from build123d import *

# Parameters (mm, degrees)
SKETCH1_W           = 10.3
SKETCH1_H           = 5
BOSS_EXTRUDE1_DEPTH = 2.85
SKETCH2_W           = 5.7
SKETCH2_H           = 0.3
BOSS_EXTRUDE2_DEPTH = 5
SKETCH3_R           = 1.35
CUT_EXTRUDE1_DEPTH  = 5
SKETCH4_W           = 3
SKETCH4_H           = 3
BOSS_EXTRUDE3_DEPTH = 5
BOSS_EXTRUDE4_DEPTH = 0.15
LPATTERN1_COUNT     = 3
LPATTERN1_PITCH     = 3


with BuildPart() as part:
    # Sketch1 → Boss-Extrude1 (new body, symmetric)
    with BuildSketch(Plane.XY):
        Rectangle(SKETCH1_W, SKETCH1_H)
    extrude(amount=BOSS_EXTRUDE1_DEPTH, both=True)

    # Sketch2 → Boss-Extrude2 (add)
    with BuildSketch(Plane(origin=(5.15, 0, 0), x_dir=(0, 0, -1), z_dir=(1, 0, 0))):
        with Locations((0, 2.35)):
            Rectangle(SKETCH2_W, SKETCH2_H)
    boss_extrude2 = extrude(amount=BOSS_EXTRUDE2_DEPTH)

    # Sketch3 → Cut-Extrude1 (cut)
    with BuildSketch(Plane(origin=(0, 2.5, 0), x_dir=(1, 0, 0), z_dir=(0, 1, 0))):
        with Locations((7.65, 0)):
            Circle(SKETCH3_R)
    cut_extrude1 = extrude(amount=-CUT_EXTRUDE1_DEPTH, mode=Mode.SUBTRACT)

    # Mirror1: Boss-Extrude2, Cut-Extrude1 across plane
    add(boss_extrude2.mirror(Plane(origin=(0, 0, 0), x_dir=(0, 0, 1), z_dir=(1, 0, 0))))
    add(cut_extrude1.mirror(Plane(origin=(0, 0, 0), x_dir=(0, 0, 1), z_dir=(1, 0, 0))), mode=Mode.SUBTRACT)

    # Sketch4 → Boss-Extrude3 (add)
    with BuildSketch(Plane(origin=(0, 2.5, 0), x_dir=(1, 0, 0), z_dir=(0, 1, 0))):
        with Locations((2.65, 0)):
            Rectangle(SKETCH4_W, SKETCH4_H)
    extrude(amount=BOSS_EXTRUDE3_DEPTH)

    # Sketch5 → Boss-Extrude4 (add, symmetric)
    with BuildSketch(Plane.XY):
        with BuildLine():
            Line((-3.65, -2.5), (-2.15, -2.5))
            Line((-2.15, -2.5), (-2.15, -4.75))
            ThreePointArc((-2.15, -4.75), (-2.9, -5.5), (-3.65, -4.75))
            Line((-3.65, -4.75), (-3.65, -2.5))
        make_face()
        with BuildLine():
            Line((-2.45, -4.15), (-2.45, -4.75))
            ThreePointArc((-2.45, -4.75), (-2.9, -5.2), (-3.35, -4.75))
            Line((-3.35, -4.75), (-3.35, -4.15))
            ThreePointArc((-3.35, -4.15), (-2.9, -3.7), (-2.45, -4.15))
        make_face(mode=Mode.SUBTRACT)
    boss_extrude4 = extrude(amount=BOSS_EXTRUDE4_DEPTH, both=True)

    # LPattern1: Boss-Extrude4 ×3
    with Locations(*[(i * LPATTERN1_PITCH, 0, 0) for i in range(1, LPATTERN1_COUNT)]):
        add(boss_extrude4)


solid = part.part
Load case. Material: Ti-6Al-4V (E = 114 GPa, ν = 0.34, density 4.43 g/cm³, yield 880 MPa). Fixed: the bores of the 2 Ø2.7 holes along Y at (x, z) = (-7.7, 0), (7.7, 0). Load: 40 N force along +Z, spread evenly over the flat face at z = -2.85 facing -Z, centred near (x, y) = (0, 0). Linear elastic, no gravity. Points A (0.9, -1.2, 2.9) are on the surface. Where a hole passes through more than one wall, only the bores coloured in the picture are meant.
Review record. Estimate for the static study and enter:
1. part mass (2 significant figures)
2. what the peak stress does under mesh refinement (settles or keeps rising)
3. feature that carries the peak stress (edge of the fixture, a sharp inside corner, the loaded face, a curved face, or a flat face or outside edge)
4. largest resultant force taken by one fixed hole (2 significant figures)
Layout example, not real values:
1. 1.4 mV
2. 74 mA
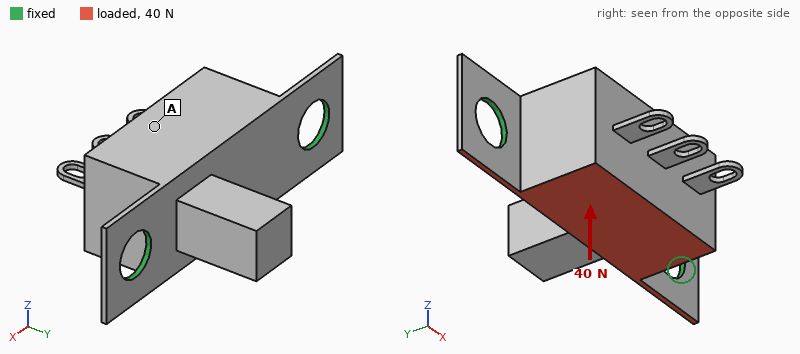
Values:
1. 1.6 g
2. keeps rising
3. edge of the fixture
4. 20 N
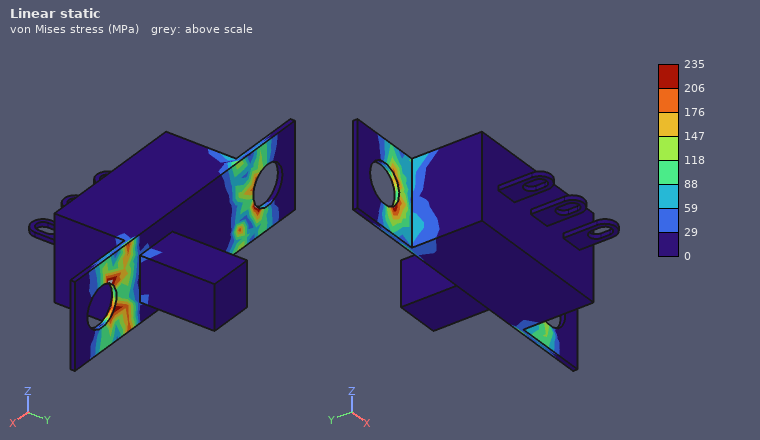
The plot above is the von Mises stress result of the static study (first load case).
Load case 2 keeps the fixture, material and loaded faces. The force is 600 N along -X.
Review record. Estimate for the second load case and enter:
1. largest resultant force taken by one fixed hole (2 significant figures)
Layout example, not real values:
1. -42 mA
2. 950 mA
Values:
1. 350 N
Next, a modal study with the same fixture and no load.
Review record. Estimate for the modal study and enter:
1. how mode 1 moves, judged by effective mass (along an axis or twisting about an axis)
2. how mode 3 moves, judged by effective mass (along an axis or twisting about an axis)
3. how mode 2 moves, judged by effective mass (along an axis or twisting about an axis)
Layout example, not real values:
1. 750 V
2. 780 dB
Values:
1. along Z
2. along X
3. along Y
